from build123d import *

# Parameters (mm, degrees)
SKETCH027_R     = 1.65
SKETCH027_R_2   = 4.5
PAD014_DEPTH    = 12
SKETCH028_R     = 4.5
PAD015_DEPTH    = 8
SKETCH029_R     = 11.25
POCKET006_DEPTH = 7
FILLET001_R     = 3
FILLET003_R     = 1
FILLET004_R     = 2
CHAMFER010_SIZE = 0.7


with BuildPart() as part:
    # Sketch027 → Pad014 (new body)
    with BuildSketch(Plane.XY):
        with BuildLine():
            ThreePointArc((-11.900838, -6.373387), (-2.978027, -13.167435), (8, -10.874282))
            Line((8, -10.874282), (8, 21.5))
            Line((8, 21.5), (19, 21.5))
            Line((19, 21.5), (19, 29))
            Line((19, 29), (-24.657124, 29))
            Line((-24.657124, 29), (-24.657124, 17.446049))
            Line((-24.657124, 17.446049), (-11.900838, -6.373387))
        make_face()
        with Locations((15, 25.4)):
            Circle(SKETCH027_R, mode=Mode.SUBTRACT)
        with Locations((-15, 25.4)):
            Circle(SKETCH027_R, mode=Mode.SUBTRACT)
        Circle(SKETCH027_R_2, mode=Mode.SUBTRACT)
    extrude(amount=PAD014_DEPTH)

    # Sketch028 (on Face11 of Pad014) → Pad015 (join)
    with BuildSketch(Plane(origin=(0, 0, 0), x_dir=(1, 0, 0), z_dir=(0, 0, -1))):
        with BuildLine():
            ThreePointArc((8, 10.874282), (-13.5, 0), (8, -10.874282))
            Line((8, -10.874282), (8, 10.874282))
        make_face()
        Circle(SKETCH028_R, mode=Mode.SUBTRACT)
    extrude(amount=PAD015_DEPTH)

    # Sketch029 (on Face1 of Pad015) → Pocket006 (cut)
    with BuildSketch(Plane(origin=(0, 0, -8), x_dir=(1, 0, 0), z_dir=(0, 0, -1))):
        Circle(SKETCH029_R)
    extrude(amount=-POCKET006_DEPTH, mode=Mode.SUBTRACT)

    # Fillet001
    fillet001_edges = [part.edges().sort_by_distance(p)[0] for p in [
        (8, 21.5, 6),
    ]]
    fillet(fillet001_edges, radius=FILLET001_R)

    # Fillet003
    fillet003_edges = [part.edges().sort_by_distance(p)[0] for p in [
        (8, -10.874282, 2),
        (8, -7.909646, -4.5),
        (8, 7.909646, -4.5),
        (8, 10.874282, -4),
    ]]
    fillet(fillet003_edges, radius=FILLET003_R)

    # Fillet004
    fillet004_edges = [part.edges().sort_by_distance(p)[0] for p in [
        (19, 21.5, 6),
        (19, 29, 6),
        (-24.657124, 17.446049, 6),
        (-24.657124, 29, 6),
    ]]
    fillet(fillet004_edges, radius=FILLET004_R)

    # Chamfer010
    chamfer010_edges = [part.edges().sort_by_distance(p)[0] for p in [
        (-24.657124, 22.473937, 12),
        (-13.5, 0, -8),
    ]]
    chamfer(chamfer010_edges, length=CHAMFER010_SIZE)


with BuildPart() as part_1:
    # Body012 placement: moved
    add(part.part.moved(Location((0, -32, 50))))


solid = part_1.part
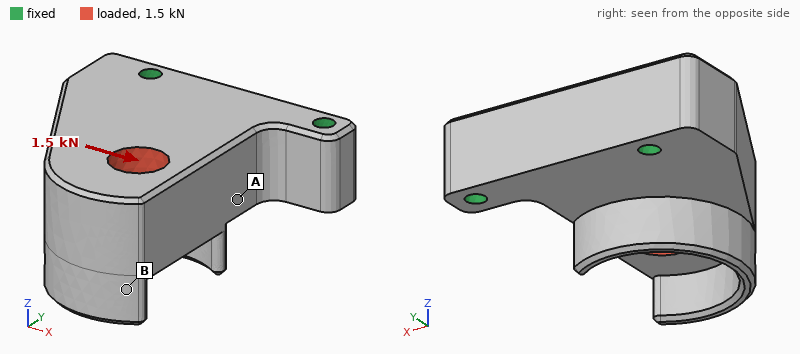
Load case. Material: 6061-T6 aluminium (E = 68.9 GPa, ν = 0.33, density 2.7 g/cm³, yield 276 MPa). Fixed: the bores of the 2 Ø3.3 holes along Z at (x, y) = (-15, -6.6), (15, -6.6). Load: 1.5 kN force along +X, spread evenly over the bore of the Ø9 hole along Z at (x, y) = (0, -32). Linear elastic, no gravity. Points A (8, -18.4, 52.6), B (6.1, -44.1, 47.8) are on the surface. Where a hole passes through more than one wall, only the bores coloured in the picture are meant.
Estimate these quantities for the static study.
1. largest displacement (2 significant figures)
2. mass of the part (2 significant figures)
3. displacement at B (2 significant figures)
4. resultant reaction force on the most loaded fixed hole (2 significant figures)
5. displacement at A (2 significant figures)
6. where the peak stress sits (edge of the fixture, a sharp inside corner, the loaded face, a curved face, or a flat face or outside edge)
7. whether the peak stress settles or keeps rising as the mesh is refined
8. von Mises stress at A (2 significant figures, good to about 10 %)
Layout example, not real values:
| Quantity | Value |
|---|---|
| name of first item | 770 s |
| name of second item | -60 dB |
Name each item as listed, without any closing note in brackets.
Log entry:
| Quantity | Value |
|---|---|
| largest displacement | 25 µm |
| mass of the part | 39 g |
| displacement at B | 25 µm |
| resultant reaction force on the most loaded fixed hole | 1.5 kN |
| displacement at A | 10 µm |
| where the peak stress sits | edge of the fixture |
| whether the peak stress settles or keeps rising as the mesh is refined | keeps rising |
| von Mises stress at A | 15 MPa |
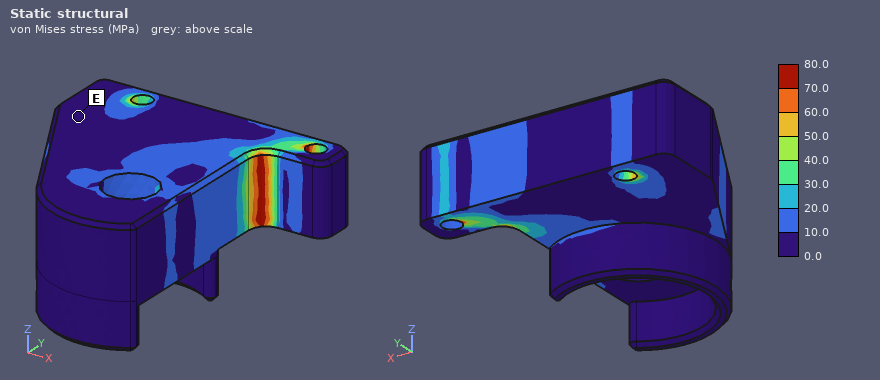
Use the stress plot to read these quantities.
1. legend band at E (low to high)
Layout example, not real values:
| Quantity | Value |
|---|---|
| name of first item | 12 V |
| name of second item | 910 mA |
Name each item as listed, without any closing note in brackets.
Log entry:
| Quantity | Value |
|---|---|
| legend band at E | 0.0 to 10.0 MPa |
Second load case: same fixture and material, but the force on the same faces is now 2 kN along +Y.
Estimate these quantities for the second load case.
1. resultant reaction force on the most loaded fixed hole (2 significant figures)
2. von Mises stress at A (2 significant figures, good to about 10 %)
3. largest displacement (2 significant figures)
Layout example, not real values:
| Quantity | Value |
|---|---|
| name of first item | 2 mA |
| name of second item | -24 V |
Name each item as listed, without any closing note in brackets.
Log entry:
| Quantity | Value |
|---|---|
| resultant reaction force on the most loaded fixed hole | 1.1 kN |
| von Mises stress at A | 16 MPa |
| largest displacement | 17 µm |
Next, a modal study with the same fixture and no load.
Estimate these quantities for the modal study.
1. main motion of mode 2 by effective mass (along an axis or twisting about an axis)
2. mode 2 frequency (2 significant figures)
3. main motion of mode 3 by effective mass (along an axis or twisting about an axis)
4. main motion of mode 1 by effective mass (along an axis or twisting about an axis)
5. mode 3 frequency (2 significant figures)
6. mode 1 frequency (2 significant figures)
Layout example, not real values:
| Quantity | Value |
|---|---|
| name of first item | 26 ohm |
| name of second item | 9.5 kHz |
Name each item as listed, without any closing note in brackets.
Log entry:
| Quantity | Value |
|---|---|
| main motion of mode 2 by effective mass | along X |
| mode 2 frequency | 9900 Hz |
| main motion of mode 3 by effective mass | twisting about Y |
| main motion of mode 1 by effective mass | along Z |
| mode 3 frequency | 17 kHz |
| mode 1 frequency | 5200 Hz |
